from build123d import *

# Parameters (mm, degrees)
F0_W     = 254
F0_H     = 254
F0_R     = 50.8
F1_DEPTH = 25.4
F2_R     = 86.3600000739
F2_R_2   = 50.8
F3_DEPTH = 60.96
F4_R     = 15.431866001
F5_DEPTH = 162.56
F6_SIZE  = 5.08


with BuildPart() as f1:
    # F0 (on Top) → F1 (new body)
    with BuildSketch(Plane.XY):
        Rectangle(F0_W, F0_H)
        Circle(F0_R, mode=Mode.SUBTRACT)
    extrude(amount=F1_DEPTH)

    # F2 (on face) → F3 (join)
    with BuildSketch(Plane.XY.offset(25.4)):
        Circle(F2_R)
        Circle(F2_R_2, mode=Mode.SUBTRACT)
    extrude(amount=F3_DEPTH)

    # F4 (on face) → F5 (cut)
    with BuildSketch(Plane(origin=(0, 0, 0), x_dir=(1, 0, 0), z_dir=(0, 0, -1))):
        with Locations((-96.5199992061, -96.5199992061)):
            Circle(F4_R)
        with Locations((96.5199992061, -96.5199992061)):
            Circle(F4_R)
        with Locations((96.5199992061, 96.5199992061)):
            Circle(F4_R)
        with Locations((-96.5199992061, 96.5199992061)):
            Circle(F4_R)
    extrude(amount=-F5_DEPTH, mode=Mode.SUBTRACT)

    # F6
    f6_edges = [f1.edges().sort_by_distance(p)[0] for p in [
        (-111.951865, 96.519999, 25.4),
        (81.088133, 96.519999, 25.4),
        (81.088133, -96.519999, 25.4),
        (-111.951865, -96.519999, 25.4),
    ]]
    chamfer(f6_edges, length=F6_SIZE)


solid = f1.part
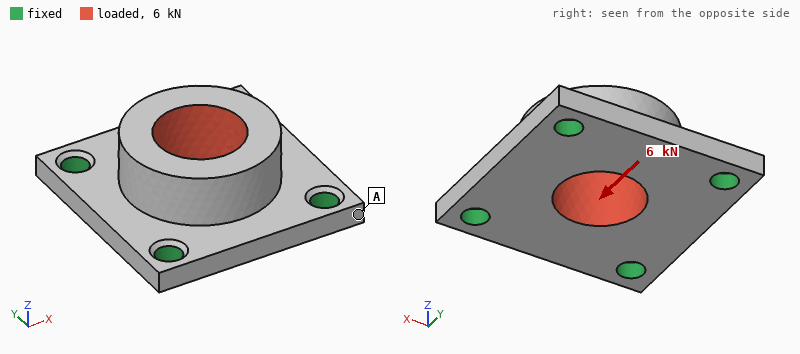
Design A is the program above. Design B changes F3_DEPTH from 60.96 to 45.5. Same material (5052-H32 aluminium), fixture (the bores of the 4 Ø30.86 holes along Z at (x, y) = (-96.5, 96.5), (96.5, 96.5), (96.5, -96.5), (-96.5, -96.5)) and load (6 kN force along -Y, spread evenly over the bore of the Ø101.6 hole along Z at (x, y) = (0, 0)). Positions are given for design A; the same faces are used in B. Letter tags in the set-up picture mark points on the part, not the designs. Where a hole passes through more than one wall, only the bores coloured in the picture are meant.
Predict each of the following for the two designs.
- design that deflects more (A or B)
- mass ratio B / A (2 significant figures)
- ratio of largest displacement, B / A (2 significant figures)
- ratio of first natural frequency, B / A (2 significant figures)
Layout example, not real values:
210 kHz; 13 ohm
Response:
A; 0.90; 0.76; 1.1
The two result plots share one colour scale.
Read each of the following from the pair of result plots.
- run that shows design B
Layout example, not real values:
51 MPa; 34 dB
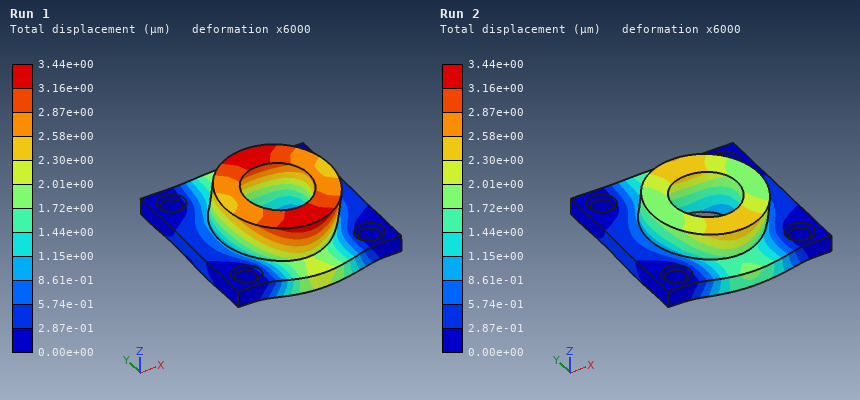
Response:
Run 2
